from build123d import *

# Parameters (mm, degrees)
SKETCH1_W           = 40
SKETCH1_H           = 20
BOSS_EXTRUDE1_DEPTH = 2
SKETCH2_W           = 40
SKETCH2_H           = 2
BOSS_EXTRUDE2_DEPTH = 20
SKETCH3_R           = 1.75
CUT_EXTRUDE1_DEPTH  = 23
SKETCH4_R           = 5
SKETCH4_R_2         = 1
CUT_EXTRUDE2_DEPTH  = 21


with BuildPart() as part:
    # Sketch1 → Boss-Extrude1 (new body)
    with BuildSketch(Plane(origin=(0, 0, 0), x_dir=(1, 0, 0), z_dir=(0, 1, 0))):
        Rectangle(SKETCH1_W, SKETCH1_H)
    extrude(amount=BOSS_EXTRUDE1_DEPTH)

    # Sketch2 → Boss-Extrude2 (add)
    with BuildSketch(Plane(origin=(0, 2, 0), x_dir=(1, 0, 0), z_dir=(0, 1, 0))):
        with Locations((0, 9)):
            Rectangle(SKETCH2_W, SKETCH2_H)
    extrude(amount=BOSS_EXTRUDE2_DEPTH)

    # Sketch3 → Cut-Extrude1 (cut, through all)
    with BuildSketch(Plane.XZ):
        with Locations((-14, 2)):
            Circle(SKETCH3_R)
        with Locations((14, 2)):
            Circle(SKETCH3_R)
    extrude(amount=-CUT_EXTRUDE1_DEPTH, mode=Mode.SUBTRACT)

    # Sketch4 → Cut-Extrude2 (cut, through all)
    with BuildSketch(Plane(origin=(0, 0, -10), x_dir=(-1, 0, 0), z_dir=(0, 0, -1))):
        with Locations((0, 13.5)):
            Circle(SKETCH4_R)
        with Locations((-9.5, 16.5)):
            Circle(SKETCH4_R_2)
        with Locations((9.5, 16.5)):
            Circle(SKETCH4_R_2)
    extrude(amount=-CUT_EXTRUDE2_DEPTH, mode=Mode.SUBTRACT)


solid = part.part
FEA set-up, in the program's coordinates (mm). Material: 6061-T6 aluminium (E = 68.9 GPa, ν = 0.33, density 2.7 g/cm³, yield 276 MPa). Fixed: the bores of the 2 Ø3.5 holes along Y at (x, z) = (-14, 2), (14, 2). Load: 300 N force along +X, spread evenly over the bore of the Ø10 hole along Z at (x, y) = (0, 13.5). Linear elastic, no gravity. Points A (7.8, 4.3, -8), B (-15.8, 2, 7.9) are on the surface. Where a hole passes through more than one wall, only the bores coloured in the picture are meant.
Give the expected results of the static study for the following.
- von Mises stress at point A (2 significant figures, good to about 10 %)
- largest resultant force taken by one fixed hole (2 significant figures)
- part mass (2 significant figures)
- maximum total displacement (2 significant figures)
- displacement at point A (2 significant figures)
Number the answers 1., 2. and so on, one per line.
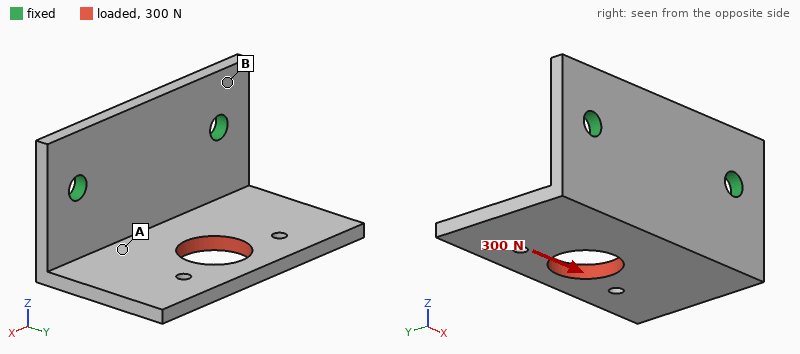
1. 29 MPa
2. 220 N
3. 8.1 g
4. 0.11 mm
5. 0.024 mm
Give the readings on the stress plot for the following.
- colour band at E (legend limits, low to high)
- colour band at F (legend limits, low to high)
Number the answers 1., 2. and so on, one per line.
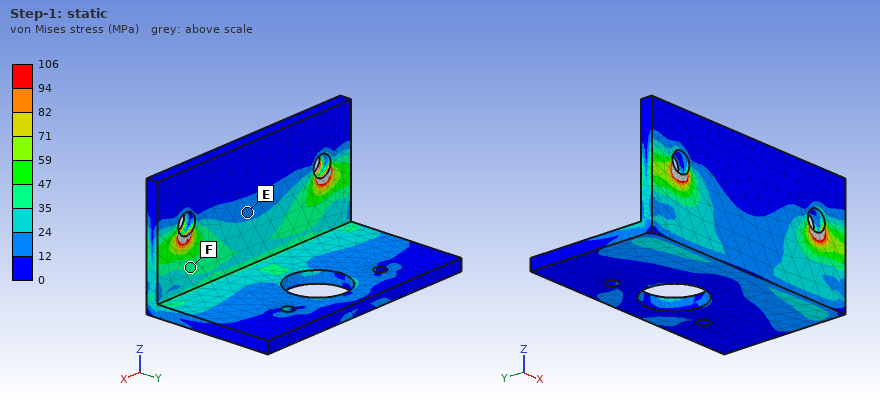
1. 12 to 24 MPa
2. 35 to 47 MPa
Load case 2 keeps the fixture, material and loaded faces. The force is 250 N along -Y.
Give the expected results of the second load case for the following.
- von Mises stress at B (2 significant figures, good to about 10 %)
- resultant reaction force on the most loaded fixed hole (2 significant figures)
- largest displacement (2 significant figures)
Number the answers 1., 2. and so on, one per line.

1. 15 MPa
2. 130 N
3. 0.19 mm
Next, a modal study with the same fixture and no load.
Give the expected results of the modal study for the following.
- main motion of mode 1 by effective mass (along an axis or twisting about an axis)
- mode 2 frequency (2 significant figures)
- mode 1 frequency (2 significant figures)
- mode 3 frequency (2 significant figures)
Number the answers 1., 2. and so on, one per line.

1. along Z
2. 3900 Hz
3. 2100 Hz
4. 6500 Hz
